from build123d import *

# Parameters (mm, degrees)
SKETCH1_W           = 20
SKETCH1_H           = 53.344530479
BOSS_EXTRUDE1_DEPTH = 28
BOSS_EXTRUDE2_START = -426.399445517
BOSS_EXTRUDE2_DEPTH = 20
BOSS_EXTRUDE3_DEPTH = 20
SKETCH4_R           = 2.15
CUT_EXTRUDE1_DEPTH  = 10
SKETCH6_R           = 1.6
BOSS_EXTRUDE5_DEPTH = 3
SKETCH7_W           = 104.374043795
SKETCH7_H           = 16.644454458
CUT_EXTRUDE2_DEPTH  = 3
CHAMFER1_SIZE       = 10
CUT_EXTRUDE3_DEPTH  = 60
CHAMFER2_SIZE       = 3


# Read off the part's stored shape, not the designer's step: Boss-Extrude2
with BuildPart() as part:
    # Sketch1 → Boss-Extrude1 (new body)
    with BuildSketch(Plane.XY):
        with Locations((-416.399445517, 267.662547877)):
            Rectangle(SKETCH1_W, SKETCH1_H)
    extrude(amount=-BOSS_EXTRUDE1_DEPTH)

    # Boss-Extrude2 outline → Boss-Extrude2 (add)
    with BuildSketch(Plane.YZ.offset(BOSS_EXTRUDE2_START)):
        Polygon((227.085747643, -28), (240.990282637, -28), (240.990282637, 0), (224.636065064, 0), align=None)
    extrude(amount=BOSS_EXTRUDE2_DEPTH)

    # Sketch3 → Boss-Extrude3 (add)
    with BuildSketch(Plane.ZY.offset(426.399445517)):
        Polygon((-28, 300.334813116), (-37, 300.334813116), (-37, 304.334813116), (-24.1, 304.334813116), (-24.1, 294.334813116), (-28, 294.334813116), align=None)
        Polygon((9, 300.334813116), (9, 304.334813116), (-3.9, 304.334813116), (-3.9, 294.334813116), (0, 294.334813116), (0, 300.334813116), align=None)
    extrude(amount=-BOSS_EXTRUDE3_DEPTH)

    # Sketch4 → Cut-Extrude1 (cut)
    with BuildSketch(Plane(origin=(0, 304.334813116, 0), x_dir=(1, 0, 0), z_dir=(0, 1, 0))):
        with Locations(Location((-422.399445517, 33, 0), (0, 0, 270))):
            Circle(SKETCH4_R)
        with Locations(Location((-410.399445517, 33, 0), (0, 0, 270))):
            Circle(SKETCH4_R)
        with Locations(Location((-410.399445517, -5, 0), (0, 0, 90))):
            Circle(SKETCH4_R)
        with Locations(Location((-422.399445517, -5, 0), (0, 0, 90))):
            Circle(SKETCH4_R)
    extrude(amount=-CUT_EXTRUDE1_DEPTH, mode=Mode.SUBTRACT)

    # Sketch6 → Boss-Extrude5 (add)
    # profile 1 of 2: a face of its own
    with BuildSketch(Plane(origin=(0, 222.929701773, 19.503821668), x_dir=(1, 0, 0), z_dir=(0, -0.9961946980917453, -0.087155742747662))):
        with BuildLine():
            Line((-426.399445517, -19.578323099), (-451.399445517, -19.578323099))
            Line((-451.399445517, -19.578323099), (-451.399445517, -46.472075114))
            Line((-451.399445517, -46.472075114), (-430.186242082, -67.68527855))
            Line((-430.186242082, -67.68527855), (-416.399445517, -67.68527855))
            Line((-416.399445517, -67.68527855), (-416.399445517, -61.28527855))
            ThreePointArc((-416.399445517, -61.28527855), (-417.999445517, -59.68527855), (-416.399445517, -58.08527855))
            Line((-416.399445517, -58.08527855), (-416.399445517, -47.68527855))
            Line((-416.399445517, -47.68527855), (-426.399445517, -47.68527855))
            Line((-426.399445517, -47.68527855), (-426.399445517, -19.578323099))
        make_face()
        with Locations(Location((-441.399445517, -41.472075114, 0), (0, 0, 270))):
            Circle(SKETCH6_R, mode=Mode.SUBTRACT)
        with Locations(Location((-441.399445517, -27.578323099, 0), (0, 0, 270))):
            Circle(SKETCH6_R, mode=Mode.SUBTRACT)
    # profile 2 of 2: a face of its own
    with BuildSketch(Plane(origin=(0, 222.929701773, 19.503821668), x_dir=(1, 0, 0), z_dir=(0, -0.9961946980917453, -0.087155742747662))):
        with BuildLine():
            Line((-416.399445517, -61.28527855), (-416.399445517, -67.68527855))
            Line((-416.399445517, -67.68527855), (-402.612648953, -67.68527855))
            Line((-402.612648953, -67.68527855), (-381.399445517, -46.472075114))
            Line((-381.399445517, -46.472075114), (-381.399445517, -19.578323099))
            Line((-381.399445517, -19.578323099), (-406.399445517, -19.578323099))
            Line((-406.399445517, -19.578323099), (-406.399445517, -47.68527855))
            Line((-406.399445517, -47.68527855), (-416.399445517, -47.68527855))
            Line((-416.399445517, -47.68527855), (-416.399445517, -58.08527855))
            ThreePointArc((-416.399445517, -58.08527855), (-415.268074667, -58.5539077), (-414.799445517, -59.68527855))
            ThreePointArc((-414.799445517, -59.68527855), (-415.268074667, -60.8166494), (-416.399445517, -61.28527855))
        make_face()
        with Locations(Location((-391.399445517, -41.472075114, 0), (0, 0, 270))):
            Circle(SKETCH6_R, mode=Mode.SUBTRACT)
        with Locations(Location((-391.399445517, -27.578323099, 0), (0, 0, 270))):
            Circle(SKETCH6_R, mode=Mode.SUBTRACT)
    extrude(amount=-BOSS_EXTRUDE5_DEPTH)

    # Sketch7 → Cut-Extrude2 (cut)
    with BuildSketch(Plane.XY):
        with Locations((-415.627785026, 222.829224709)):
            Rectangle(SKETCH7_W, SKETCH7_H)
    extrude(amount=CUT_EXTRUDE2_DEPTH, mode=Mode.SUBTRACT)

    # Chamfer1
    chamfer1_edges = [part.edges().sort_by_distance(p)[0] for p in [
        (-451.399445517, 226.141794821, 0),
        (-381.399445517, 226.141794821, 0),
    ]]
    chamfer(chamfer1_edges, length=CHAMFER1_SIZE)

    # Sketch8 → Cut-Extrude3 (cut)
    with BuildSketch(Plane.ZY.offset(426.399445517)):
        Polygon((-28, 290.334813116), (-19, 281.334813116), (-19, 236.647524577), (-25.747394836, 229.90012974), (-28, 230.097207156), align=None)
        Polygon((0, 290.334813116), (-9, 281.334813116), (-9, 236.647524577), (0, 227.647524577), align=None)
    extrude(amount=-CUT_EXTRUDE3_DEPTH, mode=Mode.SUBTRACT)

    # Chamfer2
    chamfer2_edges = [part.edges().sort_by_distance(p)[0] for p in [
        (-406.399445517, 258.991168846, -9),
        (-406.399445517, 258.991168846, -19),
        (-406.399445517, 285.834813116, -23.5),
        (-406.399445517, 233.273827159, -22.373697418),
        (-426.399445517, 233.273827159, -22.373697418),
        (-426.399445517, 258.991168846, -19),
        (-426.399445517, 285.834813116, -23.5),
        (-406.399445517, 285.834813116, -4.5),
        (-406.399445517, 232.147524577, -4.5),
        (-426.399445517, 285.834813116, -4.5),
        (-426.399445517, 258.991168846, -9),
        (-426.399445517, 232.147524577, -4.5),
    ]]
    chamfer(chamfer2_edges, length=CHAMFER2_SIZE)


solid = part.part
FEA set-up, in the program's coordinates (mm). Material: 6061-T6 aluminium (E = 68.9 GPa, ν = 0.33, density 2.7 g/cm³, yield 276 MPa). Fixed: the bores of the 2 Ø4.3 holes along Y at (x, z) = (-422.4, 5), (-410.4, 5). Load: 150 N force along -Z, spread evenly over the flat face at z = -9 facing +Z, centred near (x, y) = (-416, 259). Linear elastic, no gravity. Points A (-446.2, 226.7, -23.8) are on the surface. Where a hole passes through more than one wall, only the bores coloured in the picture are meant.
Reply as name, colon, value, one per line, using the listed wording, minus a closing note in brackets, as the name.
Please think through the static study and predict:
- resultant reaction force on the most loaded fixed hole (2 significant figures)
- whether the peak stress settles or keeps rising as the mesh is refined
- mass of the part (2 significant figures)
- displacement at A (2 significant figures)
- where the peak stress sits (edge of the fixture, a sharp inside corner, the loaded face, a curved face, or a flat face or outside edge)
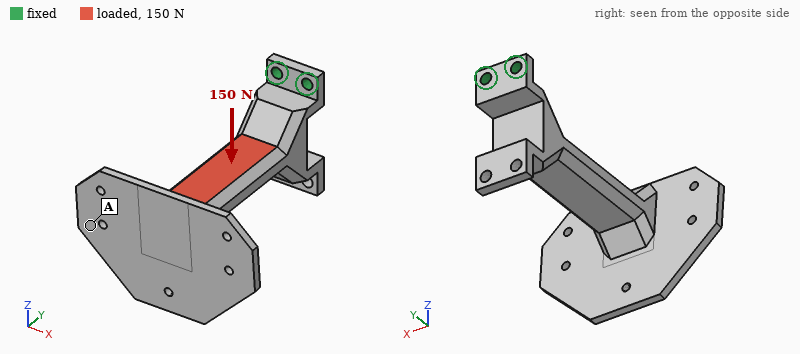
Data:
resultant reaction force on the most loaded fixed hole: 99 N
whether the peak stress settles or keeps rising as the mesh is refined: keeps rising
mass of the part: 73 g
displacement at A: 0.94 mm
where the peak stress sits: edge of the fixture
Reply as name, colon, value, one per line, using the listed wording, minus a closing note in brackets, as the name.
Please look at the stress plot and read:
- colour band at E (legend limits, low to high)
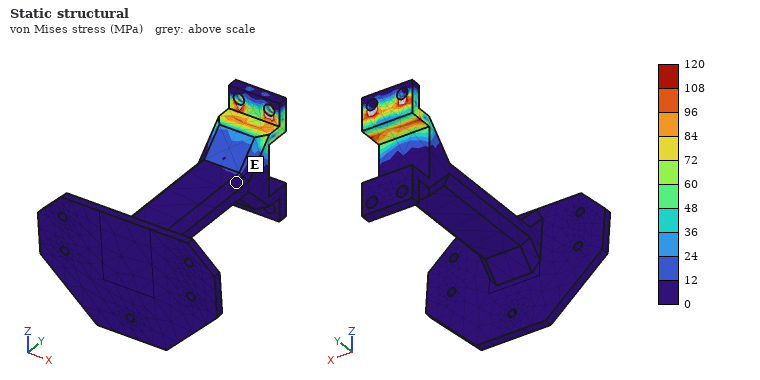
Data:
colour band at E: 0 to 12 MPa
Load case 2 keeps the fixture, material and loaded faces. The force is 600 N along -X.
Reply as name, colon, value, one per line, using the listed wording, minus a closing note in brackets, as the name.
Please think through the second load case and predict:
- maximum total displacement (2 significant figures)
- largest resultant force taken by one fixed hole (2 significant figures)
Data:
maximum total displacement: 0.55 mm
largest resultant force taken by one fixed hole: 1.9 kN
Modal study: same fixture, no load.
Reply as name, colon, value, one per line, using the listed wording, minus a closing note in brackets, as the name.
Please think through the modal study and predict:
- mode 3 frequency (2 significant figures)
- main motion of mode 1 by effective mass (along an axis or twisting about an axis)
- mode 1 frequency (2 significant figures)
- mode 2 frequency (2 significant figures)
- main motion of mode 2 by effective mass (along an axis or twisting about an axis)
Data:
mode 3 frequency: 1400 Hz
main motion of mode 1 by effective mass: along Z
mode 1 frequency: 240 Hz
mode 2 frequency: 700 Hz
main motion of mode 2 by effective mass: along X
